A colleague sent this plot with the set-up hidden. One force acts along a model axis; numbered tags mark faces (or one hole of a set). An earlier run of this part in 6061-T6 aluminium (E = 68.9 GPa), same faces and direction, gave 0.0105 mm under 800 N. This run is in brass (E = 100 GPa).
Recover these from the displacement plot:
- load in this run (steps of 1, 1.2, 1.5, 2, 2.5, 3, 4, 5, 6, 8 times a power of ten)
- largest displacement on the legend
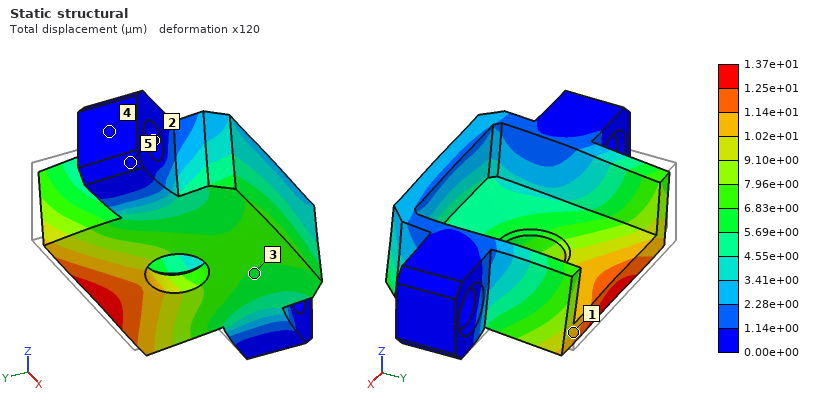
1.5 kN
1.37e+01 µm
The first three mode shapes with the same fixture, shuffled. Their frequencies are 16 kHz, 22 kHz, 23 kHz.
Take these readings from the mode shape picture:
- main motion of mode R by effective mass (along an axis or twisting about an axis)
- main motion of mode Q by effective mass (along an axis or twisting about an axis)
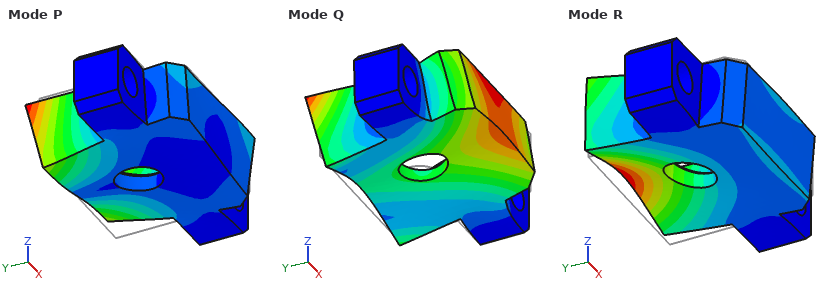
along Z
along Z
